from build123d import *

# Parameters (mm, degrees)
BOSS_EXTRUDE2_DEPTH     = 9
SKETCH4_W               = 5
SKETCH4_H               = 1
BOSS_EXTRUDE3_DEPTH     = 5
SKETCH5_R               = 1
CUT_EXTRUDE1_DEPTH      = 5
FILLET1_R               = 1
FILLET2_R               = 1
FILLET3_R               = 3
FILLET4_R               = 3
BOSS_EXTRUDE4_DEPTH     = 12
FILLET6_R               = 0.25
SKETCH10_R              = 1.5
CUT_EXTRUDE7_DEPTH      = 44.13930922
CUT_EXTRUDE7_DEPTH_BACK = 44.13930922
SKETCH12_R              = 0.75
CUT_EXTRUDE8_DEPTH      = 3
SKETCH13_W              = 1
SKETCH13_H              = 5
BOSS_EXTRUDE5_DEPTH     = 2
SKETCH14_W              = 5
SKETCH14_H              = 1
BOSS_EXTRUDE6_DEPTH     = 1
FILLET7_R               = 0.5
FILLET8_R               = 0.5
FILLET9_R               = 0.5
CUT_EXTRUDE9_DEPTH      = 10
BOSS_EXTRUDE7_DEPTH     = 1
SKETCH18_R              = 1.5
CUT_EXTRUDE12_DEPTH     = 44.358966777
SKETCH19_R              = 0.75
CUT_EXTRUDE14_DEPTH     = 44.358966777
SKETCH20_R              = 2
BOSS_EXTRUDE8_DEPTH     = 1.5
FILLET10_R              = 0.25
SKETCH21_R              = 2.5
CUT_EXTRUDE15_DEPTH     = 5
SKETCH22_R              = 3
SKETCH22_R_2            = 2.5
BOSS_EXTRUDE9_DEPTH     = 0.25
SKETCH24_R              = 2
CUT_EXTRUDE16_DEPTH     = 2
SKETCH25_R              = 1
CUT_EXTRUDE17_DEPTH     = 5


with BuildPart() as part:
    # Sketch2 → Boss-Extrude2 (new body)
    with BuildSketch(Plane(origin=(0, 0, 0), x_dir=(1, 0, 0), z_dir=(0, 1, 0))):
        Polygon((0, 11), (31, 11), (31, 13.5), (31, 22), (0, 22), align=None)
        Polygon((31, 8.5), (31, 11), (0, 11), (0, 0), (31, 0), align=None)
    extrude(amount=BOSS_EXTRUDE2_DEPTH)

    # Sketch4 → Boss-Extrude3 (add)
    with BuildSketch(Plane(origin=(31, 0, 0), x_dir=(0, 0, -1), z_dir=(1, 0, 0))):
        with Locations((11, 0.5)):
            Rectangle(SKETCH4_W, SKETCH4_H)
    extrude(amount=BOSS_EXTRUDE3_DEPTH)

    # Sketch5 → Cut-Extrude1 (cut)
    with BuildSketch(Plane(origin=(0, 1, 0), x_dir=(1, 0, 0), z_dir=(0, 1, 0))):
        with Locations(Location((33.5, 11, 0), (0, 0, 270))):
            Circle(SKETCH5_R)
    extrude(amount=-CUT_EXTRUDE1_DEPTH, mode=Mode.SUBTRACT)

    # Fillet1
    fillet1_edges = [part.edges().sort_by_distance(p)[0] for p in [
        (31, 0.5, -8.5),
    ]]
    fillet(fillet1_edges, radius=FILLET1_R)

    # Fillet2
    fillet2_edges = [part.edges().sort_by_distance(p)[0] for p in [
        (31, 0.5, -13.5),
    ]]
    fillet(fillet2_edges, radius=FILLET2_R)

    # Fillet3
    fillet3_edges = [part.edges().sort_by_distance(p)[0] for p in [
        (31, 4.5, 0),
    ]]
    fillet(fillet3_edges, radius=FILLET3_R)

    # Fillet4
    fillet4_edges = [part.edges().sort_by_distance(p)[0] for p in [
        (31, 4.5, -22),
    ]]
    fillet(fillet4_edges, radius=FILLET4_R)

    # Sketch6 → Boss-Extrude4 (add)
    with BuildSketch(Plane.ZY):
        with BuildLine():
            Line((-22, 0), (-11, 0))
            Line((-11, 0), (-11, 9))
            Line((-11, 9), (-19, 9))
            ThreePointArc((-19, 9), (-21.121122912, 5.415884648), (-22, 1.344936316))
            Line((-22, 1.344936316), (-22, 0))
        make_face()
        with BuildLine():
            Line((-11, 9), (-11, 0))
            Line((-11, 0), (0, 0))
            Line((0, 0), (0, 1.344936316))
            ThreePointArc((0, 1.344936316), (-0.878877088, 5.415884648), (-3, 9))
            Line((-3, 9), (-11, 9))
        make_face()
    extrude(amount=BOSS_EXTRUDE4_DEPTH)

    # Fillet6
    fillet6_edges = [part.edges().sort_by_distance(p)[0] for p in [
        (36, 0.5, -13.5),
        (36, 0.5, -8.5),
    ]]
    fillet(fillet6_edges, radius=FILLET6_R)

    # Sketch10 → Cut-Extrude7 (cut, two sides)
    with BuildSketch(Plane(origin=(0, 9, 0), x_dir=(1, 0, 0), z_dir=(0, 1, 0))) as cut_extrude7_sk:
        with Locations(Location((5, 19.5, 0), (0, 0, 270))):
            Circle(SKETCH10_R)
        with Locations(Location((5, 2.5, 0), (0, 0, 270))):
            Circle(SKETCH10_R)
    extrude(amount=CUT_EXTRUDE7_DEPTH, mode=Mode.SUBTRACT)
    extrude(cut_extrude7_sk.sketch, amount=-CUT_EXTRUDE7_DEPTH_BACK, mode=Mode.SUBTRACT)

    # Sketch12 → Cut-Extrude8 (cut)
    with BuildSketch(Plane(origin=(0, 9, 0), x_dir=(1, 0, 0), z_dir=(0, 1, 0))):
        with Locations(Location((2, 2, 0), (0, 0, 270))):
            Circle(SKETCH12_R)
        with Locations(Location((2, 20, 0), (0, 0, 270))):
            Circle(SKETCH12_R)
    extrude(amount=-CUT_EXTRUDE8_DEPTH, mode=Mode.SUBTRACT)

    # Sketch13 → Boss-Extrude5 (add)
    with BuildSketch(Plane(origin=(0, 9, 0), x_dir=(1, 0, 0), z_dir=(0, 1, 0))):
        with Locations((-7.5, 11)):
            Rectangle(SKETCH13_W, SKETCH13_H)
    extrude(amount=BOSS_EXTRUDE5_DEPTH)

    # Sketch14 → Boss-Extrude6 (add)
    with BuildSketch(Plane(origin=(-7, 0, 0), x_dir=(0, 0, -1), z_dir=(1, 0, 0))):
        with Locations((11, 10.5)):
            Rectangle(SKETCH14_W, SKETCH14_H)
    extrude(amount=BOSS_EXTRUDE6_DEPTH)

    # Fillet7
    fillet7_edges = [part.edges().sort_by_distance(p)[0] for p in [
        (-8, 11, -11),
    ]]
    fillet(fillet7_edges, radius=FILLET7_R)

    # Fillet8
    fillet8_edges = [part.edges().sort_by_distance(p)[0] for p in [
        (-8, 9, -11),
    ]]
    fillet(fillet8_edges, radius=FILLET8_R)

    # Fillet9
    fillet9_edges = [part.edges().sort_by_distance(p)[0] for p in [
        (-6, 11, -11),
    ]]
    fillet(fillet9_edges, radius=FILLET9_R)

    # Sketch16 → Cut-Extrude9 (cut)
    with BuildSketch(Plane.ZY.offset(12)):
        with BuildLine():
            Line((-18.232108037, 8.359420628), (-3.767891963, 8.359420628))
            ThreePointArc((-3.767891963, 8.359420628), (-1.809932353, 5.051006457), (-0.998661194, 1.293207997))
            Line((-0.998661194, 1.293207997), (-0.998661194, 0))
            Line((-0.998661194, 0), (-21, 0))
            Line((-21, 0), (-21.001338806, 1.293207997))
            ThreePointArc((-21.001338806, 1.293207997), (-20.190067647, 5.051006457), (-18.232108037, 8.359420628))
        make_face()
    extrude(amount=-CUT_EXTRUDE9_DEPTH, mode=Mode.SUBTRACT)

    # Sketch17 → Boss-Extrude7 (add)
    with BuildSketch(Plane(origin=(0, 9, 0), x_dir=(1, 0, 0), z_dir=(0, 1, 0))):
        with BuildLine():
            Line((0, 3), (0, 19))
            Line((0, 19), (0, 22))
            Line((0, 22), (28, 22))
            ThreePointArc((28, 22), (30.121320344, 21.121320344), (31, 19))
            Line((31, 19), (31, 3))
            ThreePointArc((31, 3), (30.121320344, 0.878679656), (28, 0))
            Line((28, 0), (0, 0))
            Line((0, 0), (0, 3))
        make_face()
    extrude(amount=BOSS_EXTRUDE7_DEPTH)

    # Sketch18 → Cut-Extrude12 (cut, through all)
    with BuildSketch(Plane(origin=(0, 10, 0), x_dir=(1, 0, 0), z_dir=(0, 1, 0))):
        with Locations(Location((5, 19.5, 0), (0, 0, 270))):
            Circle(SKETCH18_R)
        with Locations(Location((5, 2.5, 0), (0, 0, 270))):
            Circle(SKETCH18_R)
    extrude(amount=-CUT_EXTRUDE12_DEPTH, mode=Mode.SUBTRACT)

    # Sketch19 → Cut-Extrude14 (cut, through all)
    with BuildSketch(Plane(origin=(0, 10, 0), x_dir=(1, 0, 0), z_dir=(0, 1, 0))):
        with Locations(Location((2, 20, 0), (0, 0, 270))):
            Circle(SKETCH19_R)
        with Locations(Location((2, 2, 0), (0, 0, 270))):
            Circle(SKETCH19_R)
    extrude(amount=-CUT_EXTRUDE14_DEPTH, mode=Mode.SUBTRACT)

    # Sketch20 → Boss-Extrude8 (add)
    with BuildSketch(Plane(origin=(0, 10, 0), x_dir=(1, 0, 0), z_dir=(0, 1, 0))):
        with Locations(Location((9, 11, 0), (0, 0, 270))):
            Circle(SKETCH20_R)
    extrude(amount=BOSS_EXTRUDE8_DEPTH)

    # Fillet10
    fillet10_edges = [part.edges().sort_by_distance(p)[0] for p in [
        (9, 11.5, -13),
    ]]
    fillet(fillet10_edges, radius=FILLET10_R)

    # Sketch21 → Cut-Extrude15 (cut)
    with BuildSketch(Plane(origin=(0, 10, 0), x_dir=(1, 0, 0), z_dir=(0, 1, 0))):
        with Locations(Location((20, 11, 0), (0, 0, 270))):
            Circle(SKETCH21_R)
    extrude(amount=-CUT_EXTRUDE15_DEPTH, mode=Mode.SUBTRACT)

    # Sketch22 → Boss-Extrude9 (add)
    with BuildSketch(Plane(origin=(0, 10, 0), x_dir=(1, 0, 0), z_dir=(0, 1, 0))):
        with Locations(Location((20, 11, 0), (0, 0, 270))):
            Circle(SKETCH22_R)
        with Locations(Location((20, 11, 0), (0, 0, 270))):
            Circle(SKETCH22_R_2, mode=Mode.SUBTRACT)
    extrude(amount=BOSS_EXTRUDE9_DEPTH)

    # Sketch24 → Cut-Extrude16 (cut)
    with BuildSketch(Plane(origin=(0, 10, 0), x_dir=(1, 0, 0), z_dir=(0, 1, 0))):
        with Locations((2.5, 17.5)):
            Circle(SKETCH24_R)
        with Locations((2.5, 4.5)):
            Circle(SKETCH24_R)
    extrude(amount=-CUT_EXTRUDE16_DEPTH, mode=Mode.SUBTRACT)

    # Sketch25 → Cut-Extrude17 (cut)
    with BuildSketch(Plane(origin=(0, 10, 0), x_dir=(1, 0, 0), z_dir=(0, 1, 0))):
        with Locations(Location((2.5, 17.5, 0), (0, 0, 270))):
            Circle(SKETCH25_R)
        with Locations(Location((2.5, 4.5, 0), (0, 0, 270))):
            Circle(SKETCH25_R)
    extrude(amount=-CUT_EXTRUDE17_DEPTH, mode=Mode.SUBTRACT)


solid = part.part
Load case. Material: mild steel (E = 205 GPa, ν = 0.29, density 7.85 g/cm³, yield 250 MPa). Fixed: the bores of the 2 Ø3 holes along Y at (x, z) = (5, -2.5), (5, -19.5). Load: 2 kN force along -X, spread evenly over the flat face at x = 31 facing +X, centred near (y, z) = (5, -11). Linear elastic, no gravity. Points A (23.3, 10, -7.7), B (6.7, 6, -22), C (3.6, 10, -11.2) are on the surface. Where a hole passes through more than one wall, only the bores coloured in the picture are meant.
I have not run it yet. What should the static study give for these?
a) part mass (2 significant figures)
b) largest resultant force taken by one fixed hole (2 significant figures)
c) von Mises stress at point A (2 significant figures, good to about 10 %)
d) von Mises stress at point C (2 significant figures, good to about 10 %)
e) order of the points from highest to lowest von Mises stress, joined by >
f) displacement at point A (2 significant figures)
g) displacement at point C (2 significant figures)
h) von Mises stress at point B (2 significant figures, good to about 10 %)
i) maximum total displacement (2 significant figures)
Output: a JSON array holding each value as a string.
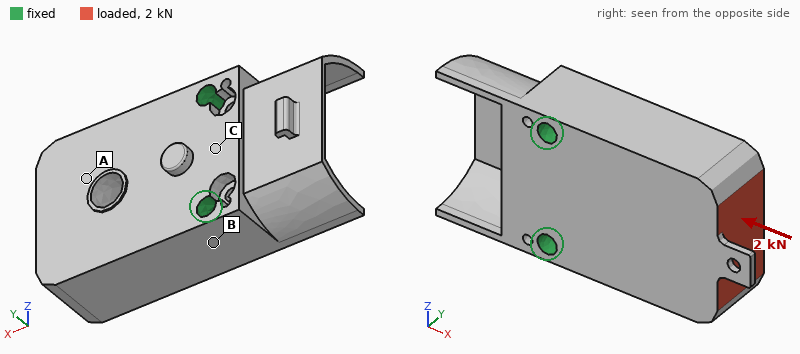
["56 g", "1.0 kN", "18 MPa", "2.6 MPa", "A > B > C", "1.3 µm", "0.38 µm", "8.0 MPa", "2.0 µm"]
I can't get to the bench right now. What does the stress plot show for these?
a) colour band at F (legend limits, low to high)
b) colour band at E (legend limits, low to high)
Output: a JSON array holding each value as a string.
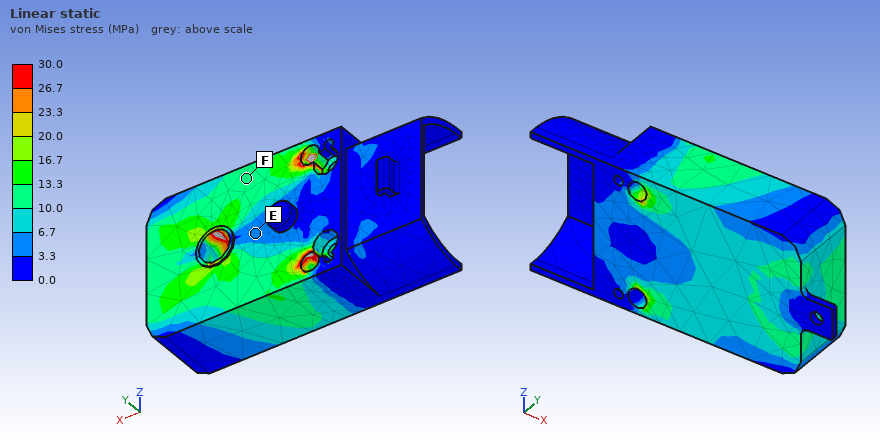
["10.0 to 13.3 MPa", "3.3 to 6.7 MPa"]
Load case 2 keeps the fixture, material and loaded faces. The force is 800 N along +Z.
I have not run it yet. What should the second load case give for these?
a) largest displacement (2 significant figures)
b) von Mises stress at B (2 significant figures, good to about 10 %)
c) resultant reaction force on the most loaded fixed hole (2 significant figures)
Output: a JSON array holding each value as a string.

["4.4 µm", "19 MPa", "1.2 kN"]
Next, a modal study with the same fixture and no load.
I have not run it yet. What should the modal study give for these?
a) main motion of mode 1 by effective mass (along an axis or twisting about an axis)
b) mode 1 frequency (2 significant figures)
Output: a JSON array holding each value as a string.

["along Y", "10 kHz"]
